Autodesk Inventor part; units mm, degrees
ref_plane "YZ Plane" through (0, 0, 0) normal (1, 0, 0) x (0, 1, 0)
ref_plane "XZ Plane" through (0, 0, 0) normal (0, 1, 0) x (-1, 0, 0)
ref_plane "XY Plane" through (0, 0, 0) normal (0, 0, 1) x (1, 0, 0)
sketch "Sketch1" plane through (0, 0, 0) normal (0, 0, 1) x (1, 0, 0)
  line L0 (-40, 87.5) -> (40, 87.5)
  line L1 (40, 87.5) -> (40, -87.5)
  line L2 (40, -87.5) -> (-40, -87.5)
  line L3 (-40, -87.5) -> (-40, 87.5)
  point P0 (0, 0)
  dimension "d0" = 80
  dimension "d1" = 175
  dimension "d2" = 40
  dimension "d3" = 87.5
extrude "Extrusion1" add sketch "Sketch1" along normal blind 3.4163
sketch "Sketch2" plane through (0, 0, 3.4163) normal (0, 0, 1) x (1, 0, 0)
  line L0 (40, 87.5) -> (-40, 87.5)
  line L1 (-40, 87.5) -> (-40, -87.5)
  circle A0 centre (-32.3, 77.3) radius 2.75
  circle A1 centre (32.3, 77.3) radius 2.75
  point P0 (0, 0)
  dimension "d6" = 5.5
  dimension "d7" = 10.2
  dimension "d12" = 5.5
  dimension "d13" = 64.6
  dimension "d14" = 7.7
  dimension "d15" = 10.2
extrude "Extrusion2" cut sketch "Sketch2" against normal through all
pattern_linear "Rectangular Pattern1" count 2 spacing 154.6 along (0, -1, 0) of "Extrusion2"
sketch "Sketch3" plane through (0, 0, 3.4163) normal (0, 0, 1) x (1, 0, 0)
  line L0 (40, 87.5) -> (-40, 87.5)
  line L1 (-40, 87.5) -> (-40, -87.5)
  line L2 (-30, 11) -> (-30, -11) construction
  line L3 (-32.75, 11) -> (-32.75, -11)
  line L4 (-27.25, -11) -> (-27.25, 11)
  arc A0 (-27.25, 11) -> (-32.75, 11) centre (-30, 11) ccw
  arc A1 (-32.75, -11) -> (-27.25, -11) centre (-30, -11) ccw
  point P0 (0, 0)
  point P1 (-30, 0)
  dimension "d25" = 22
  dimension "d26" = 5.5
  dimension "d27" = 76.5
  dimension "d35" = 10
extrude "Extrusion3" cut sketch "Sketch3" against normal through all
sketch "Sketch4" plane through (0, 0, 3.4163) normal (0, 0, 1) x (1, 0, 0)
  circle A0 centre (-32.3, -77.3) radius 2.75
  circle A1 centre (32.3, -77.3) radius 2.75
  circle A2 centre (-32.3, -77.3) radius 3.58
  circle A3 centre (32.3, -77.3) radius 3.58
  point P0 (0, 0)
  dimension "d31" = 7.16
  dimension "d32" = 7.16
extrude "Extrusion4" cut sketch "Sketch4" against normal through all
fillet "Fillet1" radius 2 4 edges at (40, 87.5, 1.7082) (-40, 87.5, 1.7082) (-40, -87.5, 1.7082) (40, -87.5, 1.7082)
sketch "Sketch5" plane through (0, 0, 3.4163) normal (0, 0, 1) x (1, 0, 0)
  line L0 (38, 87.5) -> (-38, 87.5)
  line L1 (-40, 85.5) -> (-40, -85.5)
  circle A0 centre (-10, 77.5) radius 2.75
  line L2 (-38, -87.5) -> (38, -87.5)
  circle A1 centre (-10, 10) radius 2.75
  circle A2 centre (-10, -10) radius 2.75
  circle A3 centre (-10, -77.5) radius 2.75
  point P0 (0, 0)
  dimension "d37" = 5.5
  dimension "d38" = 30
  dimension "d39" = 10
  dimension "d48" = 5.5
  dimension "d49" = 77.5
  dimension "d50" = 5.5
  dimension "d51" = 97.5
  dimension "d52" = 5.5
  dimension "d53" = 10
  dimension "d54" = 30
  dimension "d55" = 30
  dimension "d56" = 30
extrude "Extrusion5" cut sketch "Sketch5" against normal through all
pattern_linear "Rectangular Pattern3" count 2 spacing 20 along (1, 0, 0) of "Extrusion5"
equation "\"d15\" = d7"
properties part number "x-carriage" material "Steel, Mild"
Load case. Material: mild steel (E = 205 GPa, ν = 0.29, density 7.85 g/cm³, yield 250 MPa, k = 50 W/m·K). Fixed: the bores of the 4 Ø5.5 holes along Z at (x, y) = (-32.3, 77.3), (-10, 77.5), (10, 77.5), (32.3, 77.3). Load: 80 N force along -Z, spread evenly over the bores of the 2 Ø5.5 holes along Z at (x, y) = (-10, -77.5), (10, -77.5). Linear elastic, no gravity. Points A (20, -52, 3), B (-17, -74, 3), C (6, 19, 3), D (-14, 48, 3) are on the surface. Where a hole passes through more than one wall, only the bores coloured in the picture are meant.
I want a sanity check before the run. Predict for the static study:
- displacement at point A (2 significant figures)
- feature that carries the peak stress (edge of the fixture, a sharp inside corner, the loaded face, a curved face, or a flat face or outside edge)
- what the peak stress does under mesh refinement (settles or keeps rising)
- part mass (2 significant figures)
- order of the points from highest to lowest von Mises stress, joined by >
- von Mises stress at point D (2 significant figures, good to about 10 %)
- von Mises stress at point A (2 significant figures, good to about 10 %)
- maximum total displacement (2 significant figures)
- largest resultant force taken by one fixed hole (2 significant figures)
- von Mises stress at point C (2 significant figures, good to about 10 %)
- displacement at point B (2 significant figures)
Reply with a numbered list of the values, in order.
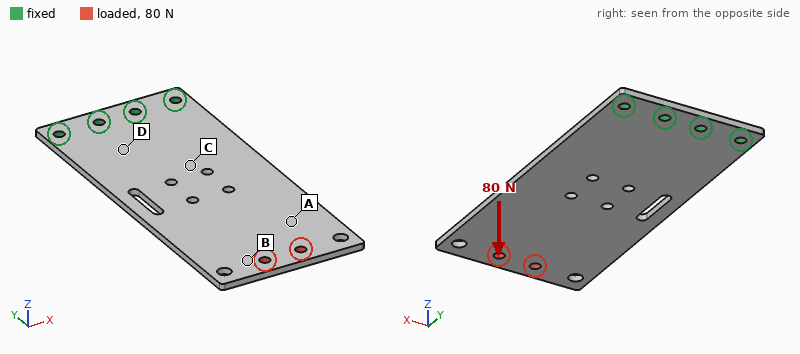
1. 1.3 mm
2. edge of the fixture
3. keeps rising
4. 360 g
5. D > C > A > B
6. 59 MPa
7. 15 MPa
8. 2.0 mm
9. 63 N
10. 46 MPa
11. 1.7 mm
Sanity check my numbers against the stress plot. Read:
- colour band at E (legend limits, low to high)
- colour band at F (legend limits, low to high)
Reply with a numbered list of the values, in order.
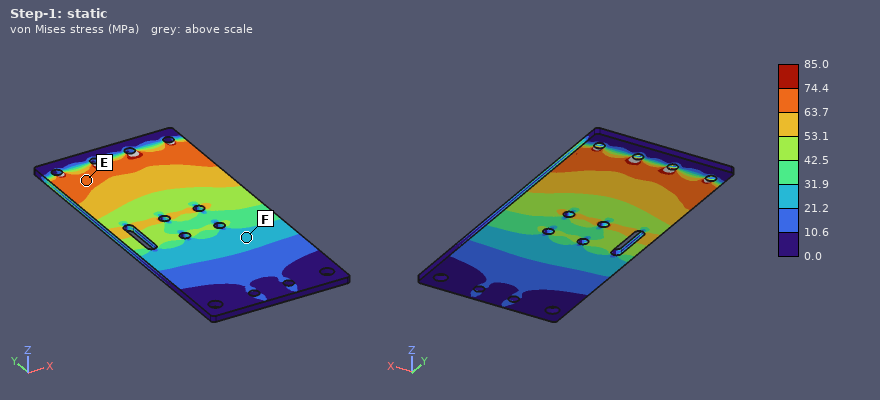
1. 63.7 to 74.4 MPa
2. 21.2 to 31.9 MPa
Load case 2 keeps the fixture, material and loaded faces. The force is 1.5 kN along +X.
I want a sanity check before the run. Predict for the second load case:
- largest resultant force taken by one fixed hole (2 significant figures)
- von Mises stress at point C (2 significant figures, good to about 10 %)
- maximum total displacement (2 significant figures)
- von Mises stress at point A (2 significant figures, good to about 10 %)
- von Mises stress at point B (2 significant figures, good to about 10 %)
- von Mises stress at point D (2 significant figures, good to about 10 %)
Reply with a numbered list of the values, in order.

1. 3.2 kN
2. 17 MPa
3. 89 µm
4. 12 MPa
5. 12 MPa
6. 22 MPa
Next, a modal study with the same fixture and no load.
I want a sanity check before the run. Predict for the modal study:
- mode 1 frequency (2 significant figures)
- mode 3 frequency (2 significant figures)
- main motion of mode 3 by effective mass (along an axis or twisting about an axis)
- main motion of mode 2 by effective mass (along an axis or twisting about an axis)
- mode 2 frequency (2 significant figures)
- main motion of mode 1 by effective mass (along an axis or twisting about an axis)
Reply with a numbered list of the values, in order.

1. 110 Hz
2. 670 Hz
3. along Z
4. twisting about Y
5. 470 Hz
6. along Z
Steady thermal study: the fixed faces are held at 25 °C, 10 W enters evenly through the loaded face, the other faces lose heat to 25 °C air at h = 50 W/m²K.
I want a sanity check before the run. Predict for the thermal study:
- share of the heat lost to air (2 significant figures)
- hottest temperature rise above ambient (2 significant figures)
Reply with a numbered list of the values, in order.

1. 97 %
2. 33 K
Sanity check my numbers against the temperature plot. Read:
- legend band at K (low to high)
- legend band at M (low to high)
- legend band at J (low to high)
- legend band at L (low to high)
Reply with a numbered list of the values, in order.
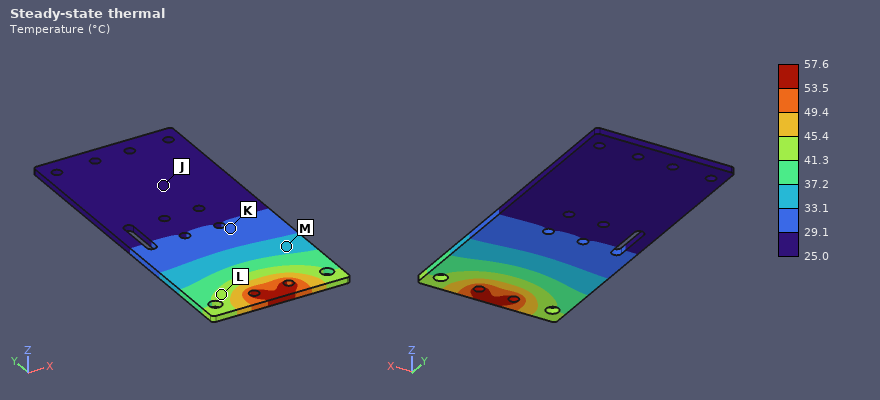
1. 29.1 to 33.1 °C
2. 33.1 to 37.2 °C
3. 25.0 to 29.1 °C
4. 41.3 to 45.4 °C
